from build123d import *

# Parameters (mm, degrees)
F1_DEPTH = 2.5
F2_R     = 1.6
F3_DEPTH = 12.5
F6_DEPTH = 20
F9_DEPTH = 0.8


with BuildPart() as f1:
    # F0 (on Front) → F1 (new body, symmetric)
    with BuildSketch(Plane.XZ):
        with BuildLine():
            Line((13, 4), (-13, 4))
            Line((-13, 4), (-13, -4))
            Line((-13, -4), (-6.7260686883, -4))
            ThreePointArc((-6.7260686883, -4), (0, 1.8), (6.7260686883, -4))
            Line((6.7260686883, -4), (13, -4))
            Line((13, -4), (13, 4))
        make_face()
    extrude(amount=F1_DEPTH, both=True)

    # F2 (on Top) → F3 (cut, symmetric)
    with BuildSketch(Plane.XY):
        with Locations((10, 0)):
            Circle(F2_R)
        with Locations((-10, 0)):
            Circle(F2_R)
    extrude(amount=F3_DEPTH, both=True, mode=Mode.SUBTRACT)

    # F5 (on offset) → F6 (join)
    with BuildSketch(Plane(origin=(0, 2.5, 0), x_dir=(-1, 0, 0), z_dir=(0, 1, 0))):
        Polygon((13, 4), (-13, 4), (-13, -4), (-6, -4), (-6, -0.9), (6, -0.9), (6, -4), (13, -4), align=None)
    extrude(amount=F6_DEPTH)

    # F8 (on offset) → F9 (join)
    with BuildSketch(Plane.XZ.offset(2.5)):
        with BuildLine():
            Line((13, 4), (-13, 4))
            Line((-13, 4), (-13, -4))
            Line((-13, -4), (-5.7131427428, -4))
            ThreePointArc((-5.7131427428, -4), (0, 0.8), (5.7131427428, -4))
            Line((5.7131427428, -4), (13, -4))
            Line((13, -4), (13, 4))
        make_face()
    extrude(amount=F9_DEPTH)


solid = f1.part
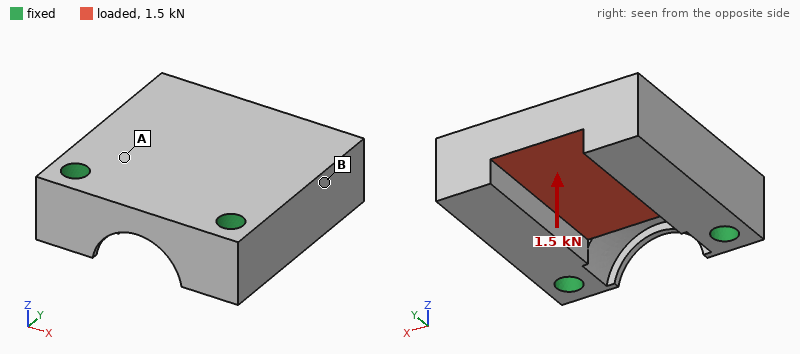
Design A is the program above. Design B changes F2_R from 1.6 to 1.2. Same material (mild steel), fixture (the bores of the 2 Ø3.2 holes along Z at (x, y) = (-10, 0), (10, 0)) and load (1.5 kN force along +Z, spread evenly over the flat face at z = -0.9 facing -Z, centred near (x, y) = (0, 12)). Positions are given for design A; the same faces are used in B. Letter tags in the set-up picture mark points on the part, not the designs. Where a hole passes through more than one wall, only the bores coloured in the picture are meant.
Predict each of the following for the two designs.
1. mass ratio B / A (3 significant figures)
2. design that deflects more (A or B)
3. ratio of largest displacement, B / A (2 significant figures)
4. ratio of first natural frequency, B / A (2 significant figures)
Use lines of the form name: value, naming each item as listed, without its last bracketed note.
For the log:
mass ratio B / A: 1.01
design that deflects more: B
ratio of largest displacement, B / A: 1.1
ratio of first natural frequency, B / A: 0.94
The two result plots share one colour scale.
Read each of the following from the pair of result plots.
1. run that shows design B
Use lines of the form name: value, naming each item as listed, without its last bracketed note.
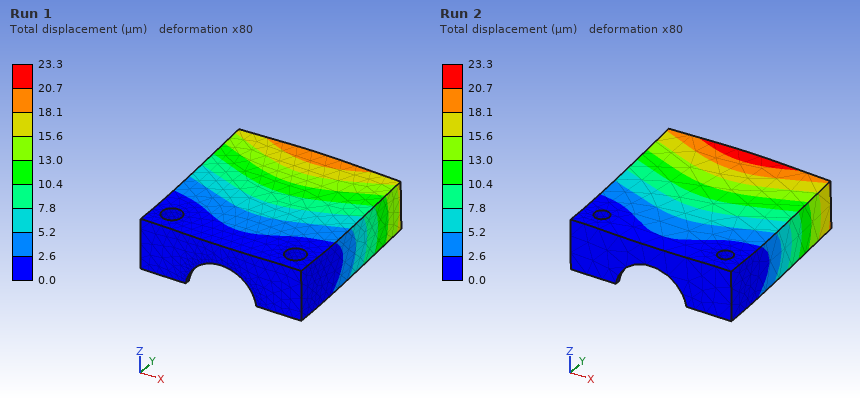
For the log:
run that shows design B: Run 2
